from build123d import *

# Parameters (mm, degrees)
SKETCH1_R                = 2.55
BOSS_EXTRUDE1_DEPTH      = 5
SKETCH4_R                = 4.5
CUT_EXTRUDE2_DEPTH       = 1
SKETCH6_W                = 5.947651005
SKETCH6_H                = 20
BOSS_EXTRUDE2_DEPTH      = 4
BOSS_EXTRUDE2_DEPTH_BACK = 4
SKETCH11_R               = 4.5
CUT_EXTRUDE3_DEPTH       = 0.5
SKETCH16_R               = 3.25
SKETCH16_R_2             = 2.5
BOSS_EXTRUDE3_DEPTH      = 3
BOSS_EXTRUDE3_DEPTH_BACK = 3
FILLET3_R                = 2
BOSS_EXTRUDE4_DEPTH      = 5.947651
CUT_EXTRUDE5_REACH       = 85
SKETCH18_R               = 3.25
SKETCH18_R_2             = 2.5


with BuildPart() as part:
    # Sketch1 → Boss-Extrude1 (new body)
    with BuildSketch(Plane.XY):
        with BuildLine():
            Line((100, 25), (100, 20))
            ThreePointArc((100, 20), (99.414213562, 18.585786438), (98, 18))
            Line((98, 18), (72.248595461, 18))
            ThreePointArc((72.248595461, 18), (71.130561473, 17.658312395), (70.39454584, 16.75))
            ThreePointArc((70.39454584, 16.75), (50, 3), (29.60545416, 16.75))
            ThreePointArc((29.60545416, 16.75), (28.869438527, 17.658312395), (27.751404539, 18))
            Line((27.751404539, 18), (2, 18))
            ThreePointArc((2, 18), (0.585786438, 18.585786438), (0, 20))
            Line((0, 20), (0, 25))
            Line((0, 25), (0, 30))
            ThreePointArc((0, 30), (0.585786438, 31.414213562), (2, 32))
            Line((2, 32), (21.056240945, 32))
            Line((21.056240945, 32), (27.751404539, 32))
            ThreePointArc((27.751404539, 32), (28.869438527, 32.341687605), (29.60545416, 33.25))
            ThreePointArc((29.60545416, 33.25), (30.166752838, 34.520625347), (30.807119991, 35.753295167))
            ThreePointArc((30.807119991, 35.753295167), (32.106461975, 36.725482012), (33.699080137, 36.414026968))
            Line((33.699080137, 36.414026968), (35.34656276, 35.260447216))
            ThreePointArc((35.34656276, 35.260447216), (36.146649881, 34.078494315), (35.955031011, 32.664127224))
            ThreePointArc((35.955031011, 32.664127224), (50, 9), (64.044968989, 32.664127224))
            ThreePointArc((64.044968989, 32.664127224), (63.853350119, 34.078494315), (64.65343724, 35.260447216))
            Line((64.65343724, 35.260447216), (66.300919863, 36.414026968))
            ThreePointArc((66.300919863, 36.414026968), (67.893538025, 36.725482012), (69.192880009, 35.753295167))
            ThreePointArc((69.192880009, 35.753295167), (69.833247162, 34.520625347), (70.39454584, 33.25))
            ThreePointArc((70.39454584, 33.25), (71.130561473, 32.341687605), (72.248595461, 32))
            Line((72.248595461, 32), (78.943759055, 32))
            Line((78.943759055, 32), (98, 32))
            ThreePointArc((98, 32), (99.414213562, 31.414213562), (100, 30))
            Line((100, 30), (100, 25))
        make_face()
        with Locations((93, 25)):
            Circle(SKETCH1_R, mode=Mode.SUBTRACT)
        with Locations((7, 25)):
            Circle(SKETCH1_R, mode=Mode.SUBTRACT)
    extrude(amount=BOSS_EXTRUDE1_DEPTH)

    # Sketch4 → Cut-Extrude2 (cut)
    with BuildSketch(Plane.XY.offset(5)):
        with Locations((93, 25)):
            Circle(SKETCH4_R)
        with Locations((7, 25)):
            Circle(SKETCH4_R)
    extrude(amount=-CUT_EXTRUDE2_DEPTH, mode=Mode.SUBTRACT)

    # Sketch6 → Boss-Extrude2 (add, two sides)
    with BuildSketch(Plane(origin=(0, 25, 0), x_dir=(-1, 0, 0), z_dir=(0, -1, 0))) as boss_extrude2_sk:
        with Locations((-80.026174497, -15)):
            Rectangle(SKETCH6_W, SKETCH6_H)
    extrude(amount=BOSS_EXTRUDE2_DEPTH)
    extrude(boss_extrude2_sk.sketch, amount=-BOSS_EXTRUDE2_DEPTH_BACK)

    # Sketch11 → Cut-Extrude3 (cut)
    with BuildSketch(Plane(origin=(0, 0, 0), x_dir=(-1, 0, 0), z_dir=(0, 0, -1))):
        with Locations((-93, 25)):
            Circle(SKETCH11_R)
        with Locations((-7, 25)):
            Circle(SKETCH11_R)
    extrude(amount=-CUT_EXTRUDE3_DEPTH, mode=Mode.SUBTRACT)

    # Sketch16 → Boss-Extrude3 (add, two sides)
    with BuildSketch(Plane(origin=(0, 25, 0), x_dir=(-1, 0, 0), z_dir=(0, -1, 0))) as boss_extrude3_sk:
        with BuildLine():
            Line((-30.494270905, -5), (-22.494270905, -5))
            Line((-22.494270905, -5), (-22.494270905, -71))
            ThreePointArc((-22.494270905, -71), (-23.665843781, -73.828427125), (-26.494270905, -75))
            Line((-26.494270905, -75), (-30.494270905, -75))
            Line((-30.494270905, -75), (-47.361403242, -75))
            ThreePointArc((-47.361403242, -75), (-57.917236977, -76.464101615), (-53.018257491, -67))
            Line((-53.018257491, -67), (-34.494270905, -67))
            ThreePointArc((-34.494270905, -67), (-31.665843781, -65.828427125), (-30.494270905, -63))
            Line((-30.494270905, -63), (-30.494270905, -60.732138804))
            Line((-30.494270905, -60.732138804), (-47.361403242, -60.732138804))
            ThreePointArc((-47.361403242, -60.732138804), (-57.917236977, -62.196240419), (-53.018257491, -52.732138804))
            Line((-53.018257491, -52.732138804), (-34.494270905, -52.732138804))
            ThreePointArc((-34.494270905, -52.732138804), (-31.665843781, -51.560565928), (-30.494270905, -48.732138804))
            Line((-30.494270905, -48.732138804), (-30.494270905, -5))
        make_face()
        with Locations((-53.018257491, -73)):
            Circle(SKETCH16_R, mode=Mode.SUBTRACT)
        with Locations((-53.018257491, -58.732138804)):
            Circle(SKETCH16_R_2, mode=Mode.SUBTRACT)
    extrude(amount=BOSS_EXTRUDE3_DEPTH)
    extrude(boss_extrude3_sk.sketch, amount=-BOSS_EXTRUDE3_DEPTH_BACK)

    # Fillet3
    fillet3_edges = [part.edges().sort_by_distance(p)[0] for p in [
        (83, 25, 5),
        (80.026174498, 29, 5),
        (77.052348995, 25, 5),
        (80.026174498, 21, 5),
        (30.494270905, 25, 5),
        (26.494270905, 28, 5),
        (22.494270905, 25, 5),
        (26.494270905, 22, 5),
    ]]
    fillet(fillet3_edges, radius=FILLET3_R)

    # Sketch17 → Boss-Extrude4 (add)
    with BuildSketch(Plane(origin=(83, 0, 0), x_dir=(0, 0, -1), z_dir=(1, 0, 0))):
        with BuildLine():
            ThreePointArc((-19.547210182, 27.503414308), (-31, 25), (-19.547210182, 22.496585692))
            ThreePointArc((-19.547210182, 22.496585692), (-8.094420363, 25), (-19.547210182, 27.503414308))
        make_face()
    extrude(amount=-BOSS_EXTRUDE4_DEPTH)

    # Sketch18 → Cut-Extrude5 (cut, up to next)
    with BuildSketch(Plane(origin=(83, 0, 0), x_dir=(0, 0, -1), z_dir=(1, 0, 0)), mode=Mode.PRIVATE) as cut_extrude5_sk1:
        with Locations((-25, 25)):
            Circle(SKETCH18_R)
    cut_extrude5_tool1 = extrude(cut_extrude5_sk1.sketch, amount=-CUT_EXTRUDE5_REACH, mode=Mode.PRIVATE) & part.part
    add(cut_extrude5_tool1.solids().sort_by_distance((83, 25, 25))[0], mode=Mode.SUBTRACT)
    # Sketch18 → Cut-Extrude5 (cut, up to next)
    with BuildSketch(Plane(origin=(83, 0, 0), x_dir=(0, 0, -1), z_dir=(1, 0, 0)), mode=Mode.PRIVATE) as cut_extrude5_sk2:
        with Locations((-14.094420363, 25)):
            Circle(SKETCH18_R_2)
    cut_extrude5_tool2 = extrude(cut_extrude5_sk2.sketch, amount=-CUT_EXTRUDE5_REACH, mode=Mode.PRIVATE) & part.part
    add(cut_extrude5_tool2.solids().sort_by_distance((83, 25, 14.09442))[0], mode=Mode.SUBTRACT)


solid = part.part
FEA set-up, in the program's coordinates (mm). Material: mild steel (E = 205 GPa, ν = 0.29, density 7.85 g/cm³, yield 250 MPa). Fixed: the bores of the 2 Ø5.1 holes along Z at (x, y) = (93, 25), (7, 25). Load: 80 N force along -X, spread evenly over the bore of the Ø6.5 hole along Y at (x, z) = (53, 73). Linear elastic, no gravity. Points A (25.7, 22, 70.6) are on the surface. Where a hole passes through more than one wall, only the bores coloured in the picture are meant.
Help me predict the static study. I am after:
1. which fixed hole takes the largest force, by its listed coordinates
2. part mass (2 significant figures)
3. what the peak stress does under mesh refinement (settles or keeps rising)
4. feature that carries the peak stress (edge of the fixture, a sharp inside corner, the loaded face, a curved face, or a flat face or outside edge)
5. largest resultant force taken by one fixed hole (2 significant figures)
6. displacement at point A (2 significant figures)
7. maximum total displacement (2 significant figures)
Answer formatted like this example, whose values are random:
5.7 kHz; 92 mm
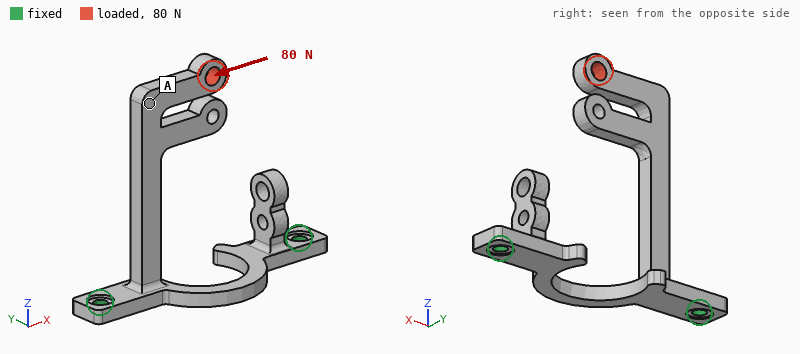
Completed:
(7, 25); 110 g; keeps rising; edge of the fixture; 92 N; 0.30 mm; 0.39 mm
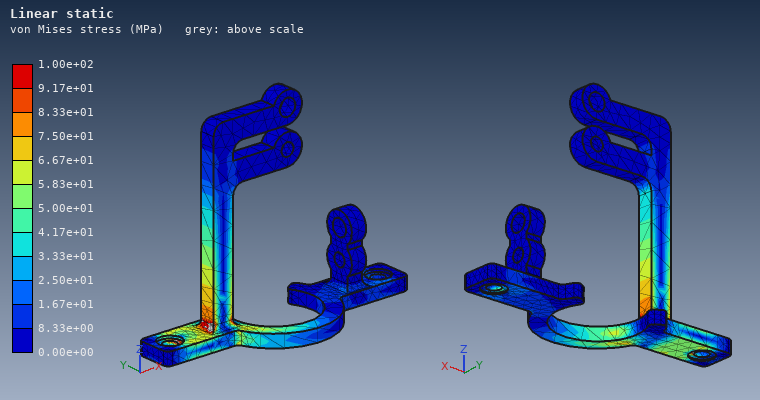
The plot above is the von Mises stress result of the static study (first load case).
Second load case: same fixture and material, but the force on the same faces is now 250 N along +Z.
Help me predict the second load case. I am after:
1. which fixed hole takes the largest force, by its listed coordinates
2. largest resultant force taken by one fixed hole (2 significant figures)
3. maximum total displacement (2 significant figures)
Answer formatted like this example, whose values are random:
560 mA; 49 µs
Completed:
(7, 25); 170 N; 0.73 mm
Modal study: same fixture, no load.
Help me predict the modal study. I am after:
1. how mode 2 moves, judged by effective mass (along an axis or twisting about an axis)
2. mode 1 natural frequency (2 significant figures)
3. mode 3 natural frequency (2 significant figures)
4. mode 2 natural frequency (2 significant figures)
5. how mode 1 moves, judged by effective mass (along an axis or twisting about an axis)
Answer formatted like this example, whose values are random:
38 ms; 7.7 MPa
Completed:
along X; 420 Hz; 1800 Hz; 480 Hz; along Y
